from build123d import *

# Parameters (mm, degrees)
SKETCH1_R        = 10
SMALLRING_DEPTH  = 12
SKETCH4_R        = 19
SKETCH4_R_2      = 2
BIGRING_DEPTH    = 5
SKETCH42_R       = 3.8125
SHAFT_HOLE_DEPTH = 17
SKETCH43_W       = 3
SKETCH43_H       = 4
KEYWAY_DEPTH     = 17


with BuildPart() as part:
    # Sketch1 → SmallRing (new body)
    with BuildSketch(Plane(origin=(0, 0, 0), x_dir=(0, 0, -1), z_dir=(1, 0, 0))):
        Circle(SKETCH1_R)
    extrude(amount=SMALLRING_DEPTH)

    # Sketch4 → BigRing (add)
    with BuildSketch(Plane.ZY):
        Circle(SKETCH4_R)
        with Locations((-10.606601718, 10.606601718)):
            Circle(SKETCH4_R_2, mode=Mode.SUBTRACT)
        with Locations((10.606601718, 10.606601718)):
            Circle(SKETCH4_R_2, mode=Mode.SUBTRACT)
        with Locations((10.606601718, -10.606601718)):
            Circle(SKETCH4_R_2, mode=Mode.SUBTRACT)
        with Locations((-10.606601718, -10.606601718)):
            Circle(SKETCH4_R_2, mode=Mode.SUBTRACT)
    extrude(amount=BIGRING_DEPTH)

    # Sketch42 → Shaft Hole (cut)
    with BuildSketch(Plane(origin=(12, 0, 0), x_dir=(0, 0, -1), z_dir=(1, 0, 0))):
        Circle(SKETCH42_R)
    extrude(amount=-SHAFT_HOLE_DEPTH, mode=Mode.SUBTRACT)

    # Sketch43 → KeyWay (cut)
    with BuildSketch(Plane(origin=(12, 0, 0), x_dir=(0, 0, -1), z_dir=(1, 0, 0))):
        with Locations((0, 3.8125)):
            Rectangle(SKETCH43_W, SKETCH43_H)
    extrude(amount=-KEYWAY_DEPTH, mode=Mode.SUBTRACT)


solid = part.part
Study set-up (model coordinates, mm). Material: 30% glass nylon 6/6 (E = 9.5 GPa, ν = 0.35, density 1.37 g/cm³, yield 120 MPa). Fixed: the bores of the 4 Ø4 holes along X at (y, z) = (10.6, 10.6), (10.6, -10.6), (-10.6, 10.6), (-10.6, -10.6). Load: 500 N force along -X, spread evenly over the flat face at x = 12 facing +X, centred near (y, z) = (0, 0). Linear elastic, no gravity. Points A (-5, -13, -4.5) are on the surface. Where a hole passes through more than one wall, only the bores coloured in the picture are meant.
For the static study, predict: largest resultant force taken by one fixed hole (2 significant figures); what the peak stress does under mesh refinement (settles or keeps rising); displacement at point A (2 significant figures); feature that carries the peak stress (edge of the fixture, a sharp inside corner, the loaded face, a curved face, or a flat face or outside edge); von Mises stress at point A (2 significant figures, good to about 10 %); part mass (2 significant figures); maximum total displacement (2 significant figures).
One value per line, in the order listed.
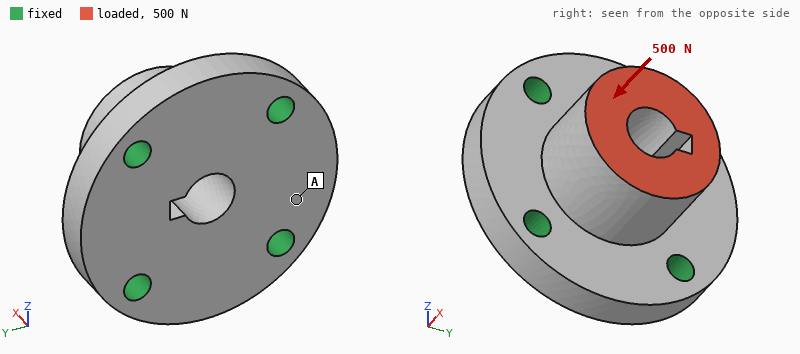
130 N
keeps rising
3.1 µm
edge of the fixture
1.7 MPa
11 g
8.9 µm
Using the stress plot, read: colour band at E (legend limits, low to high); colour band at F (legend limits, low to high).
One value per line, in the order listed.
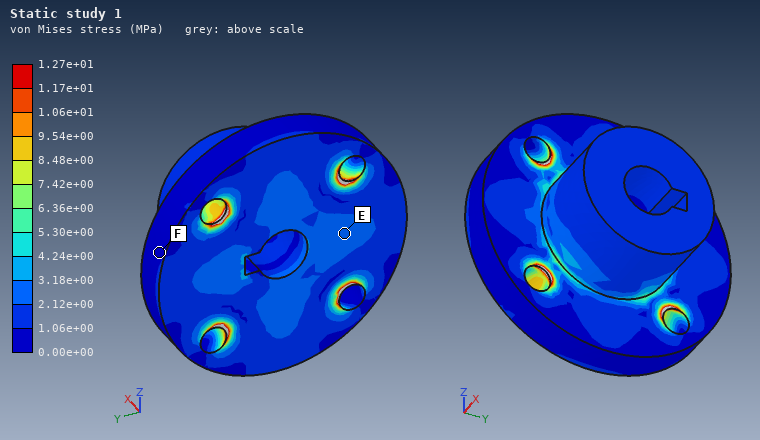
2.12e+00 to 3.18e+00 MPa
0.00e+00 to 1.06e+00 MPa
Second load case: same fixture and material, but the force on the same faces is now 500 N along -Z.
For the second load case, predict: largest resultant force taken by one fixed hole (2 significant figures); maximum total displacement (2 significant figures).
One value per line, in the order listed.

230 N
37 µm
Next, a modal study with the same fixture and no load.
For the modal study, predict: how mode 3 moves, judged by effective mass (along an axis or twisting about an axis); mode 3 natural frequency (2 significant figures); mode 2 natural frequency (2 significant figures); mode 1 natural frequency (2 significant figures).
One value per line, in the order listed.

along X
16 kHz
14 kHz
14 kHz
